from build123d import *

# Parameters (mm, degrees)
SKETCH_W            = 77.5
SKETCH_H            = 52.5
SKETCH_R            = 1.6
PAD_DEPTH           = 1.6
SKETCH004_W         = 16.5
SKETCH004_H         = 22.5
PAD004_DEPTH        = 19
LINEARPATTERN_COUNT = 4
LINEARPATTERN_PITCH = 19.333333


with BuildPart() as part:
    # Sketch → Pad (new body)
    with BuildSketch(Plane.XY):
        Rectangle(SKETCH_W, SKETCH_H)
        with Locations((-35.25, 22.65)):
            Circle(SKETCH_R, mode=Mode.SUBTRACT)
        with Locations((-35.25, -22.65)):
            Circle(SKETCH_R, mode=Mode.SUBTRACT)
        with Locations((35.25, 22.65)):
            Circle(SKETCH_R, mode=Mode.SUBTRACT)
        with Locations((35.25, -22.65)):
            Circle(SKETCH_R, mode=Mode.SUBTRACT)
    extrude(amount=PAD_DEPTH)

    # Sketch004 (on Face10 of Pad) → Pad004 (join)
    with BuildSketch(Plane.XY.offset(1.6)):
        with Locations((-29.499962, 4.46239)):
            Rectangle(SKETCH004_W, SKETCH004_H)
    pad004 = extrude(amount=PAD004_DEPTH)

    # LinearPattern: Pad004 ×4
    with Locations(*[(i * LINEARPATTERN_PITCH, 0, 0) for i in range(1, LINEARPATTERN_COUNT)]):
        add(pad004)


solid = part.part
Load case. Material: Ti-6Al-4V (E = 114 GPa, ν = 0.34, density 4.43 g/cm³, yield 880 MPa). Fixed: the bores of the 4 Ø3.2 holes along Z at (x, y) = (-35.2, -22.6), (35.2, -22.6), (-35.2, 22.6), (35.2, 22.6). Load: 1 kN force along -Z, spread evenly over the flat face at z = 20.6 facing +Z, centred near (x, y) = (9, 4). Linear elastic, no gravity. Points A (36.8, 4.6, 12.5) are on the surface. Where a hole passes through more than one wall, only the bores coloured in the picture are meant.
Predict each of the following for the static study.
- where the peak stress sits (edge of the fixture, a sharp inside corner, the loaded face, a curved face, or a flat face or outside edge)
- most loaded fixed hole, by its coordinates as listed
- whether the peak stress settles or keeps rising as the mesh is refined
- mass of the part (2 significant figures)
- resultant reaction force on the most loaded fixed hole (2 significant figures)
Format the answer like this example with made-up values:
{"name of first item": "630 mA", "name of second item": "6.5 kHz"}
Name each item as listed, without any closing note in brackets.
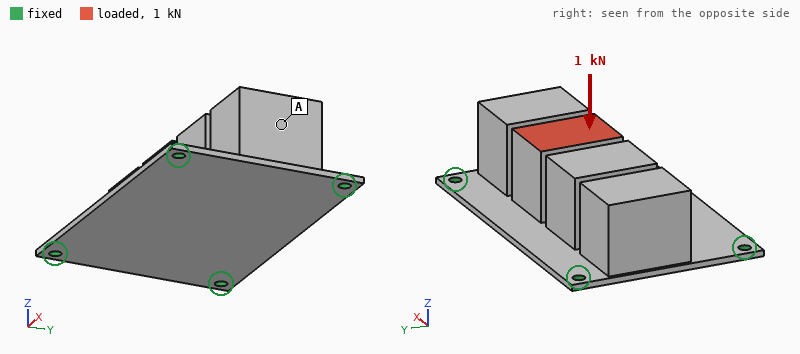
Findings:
{"where the peak stress sits": "edge of the fixture", "most loaded fixed hole, by its coordinates as listed": "(35.2, 22.6)", "whether the peak stress settles or keeps rising as the mesh is refined": "keeps rising", "mass of the part": "150 g", "resultant reaction force on the most loaded fixed hole": "510 N"}
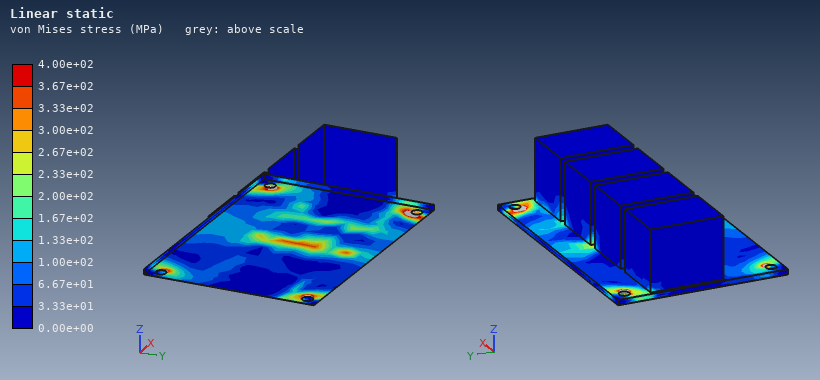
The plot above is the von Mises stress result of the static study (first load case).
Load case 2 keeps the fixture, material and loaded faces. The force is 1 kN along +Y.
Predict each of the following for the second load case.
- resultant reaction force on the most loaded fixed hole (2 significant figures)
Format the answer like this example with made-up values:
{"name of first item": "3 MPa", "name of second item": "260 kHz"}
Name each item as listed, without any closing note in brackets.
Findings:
{"resultant reaction force on the most loaded fixed hole": "480 N"}
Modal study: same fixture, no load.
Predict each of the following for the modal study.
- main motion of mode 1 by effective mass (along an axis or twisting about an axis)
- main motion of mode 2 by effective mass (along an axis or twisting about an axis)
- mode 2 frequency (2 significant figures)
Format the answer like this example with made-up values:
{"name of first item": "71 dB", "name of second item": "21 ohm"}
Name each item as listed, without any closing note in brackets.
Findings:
{"main motion of mode 1 by effective mass": "along Z", "main motion of mode 2 by effective mass": "along Y", "mode 2 frequency": "1700 Hz"}
